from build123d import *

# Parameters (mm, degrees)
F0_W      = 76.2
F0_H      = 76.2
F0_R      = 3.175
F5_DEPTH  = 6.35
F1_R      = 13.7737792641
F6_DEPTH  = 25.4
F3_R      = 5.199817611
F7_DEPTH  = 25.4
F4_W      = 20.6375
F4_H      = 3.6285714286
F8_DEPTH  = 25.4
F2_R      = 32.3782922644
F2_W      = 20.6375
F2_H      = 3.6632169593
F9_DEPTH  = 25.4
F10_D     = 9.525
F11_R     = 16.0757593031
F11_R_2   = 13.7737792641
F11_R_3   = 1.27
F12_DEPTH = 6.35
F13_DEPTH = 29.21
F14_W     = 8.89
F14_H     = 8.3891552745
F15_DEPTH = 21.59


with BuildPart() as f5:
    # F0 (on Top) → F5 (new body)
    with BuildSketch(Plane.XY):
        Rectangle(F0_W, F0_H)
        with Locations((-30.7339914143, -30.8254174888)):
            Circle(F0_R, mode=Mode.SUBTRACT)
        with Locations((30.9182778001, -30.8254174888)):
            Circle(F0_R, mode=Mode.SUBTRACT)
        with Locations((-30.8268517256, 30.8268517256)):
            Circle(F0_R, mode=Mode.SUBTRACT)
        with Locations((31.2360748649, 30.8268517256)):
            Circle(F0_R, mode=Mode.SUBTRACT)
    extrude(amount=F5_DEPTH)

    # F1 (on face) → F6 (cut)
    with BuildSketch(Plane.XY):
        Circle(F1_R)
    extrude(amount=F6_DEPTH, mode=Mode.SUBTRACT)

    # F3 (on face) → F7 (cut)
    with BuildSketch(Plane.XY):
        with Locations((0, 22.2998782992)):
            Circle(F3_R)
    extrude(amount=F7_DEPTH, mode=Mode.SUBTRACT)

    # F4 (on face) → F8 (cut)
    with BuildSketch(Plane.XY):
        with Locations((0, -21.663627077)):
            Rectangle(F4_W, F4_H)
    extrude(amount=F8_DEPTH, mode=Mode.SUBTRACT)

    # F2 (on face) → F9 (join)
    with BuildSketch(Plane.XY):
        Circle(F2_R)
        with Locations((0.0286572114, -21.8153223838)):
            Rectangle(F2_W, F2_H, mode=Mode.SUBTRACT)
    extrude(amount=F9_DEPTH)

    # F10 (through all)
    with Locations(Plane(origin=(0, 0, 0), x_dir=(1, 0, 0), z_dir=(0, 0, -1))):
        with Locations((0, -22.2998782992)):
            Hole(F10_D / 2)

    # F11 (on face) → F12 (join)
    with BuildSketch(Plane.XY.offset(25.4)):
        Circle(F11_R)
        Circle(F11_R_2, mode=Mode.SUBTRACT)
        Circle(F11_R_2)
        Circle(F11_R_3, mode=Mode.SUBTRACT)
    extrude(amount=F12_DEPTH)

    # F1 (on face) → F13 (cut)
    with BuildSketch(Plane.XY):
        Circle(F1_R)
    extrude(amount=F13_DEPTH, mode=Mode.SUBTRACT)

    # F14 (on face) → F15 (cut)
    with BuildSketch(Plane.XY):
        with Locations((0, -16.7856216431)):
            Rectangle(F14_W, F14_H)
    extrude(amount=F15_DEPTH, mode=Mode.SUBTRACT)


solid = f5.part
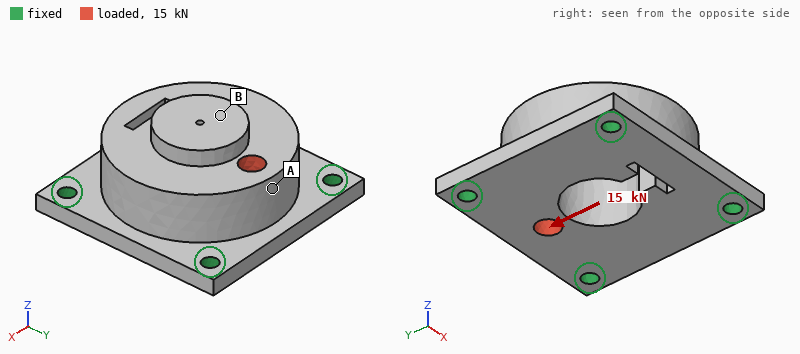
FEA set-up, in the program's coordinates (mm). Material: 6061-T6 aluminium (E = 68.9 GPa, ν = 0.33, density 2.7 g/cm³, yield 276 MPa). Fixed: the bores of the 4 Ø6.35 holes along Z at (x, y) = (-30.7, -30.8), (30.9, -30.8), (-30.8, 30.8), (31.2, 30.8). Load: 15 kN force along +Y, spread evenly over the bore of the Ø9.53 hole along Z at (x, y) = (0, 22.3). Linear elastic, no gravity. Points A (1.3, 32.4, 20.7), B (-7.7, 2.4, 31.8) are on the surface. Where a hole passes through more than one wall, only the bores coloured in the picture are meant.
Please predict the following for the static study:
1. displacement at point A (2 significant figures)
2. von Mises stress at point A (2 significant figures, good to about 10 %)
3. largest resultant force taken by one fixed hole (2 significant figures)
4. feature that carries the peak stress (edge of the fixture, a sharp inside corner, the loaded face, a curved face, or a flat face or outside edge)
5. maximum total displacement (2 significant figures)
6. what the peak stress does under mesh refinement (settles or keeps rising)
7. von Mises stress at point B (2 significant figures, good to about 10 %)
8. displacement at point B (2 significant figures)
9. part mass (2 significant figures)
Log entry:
37 µm
47 MPa
4.3 kN
edge of the fixture
40 µm
keeps rising
11 MPa
26 µm
220 g
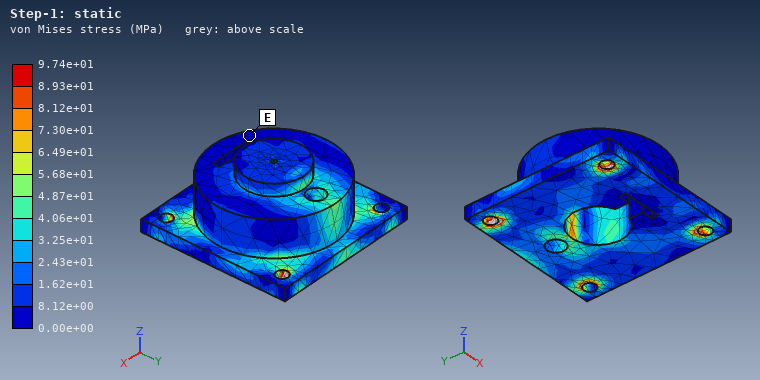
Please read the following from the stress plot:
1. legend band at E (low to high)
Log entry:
0.00e+00 to 8.12e+00 MPa
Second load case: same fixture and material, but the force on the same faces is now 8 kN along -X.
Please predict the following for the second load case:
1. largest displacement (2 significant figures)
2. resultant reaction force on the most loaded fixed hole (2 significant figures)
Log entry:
18 µm
3.4 kN
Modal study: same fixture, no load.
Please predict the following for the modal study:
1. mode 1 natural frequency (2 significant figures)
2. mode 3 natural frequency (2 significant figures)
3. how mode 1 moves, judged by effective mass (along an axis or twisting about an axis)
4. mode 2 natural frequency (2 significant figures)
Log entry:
6700 Hz
8200 Hz
along Z
7900 Hz
